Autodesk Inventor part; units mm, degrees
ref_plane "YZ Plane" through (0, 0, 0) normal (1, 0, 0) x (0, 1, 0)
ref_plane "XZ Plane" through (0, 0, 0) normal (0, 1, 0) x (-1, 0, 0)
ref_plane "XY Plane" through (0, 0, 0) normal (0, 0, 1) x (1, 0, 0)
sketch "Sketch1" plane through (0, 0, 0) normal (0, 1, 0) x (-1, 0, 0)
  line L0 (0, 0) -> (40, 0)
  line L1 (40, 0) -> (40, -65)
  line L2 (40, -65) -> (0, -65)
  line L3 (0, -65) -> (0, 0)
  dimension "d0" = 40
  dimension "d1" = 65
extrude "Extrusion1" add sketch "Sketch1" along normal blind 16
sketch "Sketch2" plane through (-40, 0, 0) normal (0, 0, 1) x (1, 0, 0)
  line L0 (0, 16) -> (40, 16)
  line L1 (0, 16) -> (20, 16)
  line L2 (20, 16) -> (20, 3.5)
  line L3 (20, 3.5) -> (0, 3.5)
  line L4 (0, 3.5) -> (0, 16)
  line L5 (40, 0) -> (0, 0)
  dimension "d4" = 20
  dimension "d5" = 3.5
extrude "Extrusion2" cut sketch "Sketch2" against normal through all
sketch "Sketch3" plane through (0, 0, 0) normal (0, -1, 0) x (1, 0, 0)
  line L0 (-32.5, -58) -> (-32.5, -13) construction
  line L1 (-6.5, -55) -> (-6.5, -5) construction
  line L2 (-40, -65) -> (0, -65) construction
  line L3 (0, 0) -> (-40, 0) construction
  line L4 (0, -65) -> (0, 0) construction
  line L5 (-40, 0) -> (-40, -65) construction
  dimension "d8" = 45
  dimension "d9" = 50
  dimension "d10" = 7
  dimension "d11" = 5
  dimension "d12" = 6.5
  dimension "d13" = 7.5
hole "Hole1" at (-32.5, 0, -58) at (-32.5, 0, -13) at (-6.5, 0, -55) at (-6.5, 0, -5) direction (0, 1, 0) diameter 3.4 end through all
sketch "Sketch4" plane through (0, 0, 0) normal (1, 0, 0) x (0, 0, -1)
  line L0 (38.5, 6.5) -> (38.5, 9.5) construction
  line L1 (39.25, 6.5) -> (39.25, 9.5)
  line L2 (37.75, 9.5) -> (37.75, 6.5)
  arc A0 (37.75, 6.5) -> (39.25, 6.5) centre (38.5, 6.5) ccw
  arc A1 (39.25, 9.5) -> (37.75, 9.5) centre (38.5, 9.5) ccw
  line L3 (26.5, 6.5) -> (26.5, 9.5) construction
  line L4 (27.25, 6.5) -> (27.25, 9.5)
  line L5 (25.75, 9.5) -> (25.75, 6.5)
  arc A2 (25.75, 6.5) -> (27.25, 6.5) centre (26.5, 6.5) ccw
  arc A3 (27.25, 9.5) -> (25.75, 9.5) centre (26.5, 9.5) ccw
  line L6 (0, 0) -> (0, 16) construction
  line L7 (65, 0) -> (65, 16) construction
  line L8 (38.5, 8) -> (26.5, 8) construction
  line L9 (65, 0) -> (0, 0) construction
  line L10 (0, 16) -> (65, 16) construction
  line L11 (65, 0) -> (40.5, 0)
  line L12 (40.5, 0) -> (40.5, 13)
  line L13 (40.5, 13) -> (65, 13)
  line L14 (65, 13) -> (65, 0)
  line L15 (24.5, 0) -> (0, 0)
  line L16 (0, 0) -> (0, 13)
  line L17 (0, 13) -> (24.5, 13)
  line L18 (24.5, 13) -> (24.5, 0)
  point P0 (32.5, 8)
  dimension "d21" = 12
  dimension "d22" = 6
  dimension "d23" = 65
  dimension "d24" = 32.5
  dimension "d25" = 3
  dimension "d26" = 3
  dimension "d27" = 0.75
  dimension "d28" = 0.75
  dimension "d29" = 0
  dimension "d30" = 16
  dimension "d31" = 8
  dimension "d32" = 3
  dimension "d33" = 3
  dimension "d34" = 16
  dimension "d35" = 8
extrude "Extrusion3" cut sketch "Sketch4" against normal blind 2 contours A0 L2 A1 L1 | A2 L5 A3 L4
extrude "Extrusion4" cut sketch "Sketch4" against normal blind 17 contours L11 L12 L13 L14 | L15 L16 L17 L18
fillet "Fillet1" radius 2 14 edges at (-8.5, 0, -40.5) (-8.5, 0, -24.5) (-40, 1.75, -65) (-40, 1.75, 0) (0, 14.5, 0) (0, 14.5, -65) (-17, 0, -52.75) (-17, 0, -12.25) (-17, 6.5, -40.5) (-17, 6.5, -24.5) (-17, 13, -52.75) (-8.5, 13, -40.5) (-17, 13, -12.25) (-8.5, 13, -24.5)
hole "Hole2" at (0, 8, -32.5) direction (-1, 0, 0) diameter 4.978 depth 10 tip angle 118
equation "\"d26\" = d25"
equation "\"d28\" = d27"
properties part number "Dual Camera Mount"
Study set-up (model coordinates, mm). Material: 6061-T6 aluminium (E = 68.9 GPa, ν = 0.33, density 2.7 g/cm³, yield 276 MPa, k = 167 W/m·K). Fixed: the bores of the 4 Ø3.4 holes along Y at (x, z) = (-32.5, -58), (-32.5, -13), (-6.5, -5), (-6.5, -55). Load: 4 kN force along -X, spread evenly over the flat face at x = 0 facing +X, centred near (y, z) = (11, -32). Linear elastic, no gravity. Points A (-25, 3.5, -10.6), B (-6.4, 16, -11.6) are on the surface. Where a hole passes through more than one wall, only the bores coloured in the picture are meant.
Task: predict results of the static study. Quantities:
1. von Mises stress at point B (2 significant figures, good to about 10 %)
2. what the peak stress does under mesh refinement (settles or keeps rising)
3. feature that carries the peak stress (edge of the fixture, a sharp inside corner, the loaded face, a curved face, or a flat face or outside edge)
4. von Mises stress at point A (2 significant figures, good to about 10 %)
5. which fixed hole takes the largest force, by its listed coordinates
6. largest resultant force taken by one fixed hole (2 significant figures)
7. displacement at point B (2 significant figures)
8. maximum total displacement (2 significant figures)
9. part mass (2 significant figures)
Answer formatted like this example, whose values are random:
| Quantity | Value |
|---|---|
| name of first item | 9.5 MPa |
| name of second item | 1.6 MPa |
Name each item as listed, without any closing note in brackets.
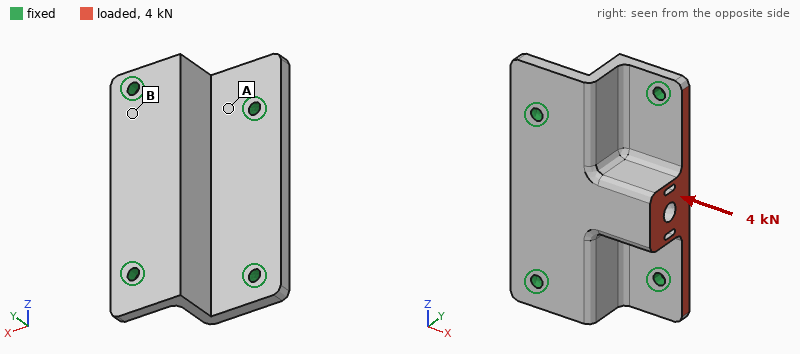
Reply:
| Quantity | Value |
|---|---|
| von Mises stress at point B | 34 MPa |
| what the peak stress does under mesh refinement | keeps rising |
| feature that carries the peak stress | edge of the fixture |
| von Mises stress at point A | 13 MPa |
| which fixed hole takes the largest force, by its listed coordinates | (-6.5, -55) |
| largest resultant force taken by one fixed hole | 1.5 kN |
| displacement at point B | 9.8 µm |
| maximum total displacement | 29 µm |
| part mass | 38 g |
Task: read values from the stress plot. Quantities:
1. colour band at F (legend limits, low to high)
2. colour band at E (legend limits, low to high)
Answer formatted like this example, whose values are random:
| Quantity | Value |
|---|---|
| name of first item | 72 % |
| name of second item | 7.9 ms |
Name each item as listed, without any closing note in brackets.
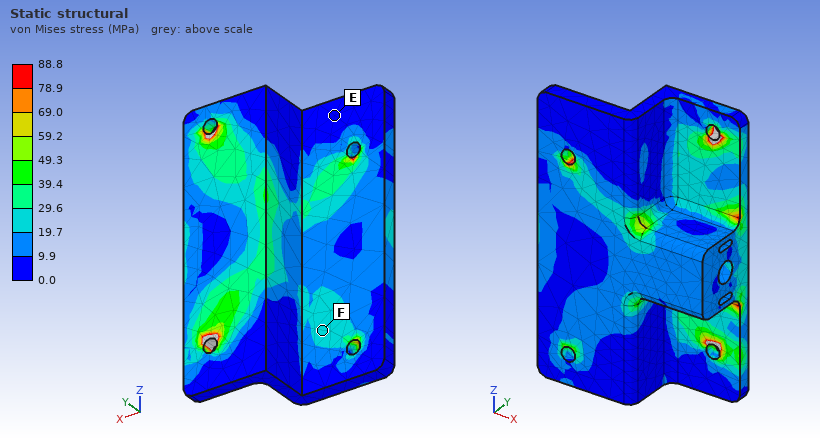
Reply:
| Quantity | Value |
|---|---|
| colour band at F | 19.7 to 29.6 MPa |
| colour band at E | 0.0 to 9.9 MPa |
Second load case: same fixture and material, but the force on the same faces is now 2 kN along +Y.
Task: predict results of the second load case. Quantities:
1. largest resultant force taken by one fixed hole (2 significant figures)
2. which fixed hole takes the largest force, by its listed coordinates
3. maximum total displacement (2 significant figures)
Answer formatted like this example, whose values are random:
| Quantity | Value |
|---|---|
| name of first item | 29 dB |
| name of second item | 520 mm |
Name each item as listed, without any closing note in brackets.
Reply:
| Quantity | Value |
|---|---|
| largest resultant force taken by one fixed hole | 1.2 kN |
| which fixed hole takes the largest force, by its listed coordinates | (-6.5, -55) |
| maximum total displacement | 94 µm |
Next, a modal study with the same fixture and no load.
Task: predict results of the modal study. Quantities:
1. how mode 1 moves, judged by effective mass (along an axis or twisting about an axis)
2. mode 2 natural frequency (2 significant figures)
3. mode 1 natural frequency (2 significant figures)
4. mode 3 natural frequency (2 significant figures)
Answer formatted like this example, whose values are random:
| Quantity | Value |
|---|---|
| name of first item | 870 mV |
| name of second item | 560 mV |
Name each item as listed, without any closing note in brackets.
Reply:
| Quantity | Value |
|---|---|
| how mode 1 moves, judged by effective mass | along Y |
| mode 2 natural frequency | 11 kHz |
| mode 1 natural frequency | 6600 Hz |
| mode 3 natural frequency | 14 kHz |
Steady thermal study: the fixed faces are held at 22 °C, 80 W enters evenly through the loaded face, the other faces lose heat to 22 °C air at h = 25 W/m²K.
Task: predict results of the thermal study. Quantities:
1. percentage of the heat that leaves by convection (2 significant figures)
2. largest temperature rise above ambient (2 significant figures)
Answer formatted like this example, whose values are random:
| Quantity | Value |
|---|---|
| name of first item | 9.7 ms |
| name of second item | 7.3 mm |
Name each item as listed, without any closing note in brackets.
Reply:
| Quantity | Value |
|---|---|
| percentage of the heat that leaves by convection | 3.9 % |
| largest temperature rise above ambient | 45 K |
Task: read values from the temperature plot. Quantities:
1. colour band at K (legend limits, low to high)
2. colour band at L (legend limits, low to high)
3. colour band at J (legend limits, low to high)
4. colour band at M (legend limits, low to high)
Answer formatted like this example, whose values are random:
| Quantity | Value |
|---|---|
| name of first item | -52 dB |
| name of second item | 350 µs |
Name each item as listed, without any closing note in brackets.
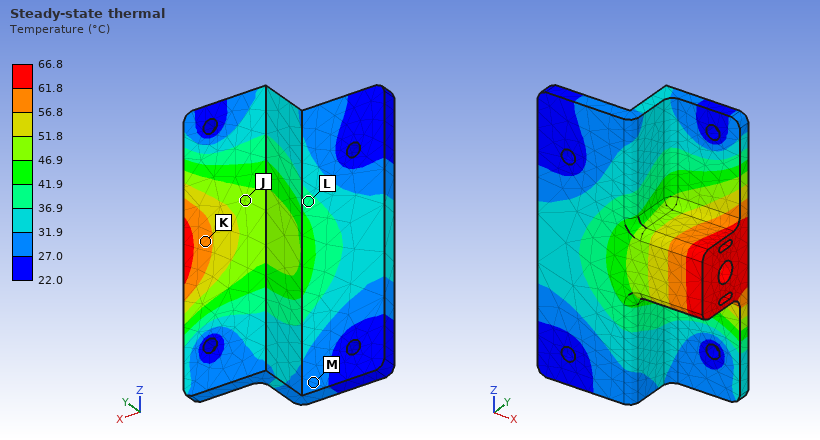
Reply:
| Quantity | Value |
|---|---|
| colour band at K | 56.8 to 61.8 °C |
| colour band at L | 36.9 to 41.9 °C |
| colour band at J | 46.9 to 51.8 °C |
| colour band at M | 27.0 to 31.9 °C |
